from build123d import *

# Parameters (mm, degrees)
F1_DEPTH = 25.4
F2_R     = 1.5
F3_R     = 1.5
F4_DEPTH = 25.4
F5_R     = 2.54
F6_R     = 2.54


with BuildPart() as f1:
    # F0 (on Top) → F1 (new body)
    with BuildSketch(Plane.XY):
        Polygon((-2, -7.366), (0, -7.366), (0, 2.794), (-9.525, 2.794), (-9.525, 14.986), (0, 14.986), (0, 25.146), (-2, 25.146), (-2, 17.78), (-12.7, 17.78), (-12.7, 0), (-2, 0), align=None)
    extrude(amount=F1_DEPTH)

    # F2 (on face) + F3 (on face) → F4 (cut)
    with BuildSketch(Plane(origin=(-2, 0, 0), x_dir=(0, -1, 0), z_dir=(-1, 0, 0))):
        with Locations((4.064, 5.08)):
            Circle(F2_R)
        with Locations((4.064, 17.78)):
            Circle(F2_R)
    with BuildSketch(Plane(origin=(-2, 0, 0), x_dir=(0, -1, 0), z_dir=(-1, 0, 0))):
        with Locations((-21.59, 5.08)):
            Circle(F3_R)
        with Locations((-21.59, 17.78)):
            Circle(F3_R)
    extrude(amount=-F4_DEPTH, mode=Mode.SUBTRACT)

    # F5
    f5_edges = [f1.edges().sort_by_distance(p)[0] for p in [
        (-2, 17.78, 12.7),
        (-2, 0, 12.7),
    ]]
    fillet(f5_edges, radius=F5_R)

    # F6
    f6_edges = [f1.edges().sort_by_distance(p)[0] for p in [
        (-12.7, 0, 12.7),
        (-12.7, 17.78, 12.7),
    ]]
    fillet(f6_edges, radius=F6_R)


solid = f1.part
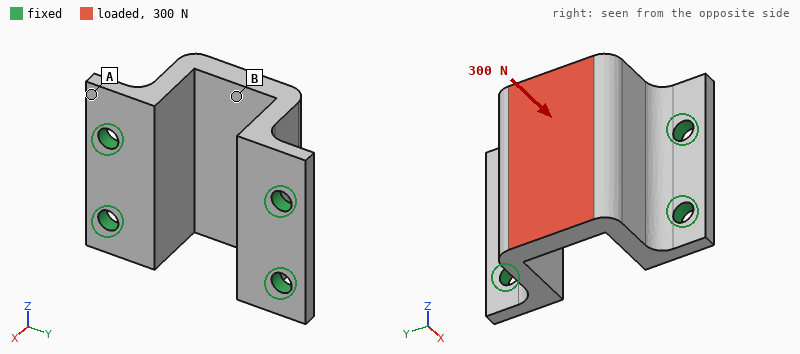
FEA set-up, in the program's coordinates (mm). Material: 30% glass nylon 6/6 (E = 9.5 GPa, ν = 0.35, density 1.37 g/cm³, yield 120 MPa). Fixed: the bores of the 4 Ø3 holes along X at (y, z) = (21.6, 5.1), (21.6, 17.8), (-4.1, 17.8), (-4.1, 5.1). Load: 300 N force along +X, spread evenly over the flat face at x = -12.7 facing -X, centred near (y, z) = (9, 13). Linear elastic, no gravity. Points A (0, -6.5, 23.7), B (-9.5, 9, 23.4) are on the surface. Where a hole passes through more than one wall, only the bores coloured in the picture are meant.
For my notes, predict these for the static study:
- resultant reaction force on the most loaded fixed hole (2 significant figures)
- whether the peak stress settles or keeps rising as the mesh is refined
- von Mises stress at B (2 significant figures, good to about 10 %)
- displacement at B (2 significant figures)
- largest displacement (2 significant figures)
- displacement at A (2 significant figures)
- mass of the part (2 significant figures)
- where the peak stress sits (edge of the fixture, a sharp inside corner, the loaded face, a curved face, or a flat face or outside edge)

100 N
keeps rising
4.8 MPa
23 µm
25 µm
4.0 µm
4.8 g
edge of the fixture
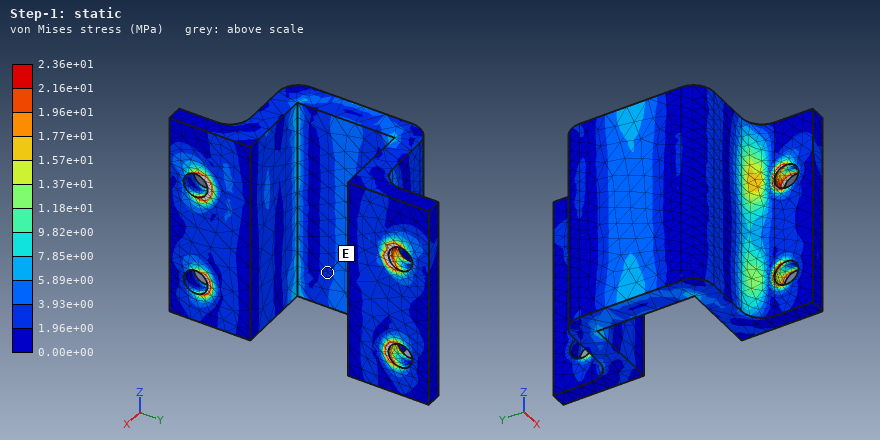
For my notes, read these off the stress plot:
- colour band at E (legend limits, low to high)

1.96e+00 to 3.93e+00 MPa
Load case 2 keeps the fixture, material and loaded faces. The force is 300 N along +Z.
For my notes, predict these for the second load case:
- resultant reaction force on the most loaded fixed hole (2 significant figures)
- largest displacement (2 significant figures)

170 N
64 µm
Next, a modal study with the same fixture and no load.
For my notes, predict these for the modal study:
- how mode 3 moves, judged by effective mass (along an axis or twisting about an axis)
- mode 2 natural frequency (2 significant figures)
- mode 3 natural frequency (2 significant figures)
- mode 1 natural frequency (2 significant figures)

twisting about X
7700 Hz
9400 Hz
7700 Hz
